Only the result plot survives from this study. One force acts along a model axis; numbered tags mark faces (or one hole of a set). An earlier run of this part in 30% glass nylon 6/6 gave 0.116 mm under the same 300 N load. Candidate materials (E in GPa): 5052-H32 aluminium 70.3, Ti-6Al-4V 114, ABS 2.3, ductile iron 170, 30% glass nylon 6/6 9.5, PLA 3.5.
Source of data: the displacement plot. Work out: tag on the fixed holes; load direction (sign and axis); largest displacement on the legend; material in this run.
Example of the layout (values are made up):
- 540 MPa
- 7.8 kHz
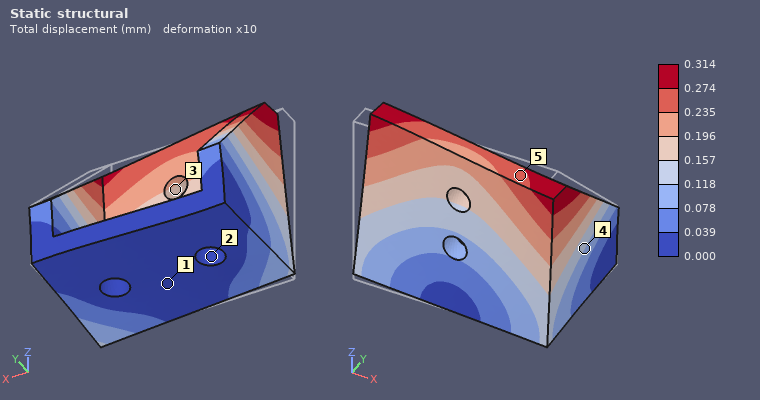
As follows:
- 2
- +X
- 0.314 mm
- PLA
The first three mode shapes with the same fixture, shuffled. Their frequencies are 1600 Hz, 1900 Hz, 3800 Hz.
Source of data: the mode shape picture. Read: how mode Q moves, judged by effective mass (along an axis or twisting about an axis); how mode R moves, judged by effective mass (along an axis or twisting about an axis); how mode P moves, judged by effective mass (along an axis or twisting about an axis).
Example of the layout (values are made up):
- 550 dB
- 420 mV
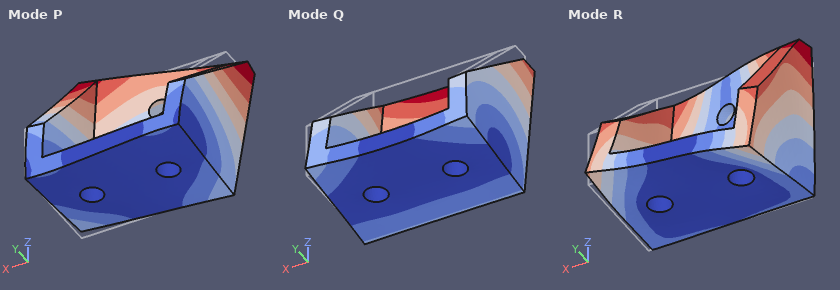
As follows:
- along Y
- along X
- along X
